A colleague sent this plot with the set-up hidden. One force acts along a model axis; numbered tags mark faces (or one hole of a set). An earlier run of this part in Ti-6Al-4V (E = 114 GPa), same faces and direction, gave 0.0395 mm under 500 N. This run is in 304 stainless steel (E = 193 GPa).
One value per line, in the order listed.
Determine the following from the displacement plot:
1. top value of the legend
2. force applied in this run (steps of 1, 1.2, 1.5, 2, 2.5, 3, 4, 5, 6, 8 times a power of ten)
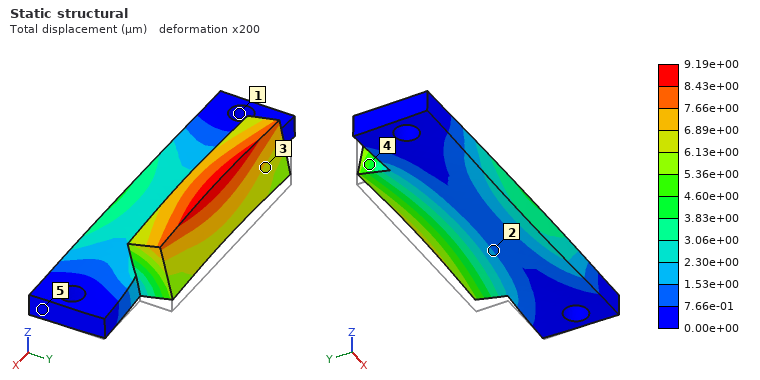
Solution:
9.19e+00 µm
200 N
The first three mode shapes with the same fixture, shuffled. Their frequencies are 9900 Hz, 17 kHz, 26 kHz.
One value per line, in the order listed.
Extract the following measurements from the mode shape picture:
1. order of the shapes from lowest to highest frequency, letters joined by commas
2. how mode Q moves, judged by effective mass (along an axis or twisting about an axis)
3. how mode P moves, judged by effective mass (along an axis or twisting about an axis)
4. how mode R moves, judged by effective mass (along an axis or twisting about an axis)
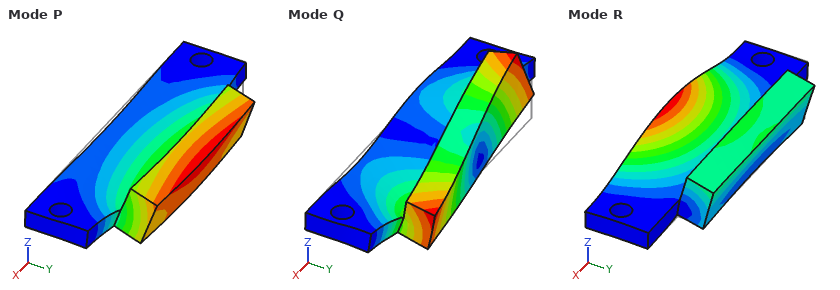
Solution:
P, R, Q
twisting about Y
along Z
along Z
